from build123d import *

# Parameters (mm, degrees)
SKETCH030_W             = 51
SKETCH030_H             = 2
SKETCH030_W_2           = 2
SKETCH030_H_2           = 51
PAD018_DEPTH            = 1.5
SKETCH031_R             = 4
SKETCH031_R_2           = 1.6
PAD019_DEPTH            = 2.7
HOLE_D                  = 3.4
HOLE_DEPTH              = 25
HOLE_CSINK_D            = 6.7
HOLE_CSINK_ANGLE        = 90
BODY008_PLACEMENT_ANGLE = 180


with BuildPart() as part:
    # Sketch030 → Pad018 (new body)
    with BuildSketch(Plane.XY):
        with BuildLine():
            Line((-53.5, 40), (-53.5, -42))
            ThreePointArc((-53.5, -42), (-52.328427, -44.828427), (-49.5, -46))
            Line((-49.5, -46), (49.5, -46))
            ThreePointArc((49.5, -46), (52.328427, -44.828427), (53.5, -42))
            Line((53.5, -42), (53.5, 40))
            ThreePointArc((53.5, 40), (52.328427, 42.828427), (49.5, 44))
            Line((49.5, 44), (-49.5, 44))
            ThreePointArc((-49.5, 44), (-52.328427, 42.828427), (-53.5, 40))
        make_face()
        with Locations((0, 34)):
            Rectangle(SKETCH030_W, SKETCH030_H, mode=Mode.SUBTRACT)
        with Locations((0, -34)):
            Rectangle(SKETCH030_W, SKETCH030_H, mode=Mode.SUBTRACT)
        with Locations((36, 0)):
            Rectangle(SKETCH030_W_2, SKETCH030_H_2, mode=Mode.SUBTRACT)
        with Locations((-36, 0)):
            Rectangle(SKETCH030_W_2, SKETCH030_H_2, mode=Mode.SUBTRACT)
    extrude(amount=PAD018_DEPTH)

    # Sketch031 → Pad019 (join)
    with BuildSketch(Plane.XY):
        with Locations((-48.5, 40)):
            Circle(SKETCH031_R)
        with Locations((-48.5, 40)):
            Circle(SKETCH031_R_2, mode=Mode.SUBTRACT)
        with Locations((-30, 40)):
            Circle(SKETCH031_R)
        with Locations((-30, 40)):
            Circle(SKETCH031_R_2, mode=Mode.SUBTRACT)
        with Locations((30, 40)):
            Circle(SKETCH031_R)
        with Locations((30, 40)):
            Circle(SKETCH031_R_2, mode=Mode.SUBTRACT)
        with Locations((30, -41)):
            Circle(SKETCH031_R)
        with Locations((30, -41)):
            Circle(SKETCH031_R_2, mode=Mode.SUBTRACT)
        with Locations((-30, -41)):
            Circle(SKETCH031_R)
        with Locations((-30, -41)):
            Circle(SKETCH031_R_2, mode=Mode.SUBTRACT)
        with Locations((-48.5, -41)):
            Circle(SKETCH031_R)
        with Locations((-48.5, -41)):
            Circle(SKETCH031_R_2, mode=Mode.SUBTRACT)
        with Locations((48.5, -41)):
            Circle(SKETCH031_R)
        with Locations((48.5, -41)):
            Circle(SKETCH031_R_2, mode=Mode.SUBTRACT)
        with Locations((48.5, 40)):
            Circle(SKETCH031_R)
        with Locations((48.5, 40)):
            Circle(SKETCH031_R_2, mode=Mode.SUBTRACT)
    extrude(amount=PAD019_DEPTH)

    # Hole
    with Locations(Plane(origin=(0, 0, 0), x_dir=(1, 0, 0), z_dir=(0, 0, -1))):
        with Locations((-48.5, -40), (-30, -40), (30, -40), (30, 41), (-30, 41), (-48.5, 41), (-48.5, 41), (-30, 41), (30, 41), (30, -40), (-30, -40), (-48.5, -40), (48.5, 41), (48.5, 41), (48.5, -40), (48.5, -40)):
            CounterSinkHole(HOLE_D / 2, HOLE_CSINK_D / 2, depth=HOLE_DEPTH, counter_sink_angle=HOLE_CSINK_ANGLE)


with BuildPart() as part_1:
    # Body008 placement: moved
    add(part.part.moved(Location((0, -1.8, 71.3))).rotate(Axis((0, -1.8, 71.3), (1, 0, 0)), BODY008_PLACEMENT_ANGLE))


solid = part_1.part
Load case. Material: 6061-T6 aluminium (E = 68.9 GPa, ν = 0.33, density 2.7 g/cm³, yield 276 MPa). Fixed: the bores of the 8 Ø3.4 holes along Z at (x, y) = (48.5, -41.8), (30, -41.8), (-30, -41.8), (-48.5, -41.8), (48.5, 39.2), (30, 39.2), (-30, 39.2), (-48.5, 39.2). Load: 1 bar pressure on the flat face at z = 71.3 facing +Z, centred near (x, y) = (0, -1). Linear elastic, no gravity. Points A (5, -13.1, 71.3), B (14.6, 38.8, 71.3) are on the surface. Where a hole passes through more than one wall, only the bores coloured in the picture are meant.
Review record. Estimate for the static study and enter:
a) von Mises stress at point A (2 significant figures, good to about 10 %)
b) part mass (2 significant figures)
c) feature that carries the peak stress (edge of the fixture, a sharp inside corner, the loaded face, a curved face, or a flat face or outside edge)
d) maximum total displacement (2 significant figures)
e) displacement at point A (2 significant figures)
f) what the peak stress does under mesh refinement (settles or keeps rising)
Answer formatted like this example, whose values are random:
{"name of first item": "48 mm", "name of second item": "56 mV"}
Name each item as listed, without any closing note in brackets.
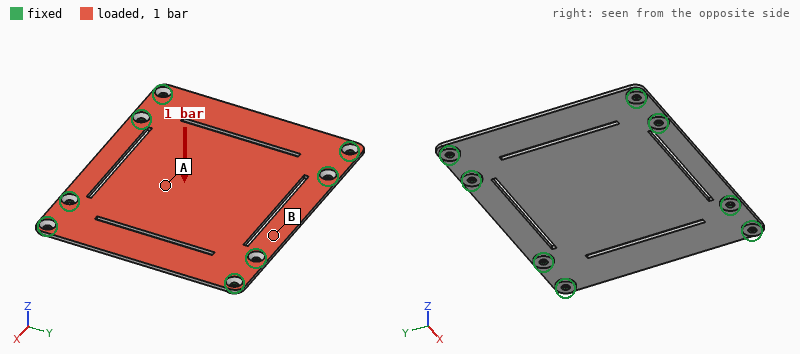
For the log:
{"von Mises stress at point A": "72 MPa", "part mass": "38 g", "feature that carries the peak stress": "edge of the fixture", "maximum total displacement": "0.97 mm", "displacement at point A": "0.88 mm", "what the peak stress does under mesh refinement": "keeps rising"}
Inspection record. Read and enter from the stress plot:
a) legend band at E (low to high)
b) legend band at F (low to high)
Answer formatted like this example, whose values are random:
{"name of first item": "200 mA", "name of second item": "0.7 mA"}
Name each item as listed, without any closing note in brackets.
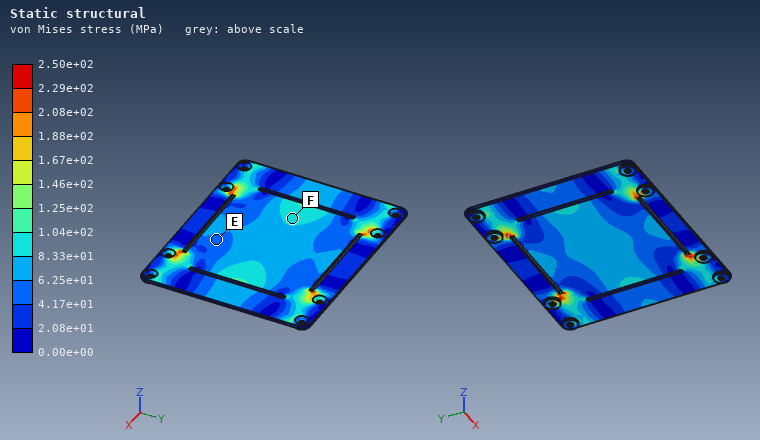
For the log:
{"legend band at E": "4.17e+01 to 6.25e+01 MPa", "legend band at F": "8.33e+01 to 1.04e+02 MPa"}
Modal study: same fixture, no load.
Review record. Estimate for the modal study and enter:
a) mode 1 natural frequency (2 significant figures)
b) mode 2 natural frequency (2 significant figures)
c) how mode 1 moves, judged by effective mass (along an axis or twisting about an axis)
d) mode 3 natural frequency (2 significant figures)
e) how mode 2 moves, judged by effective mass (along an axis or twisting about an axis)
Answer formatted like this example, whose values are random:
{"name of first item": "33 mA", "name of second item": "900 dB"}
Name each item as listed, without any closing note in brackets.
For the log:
{"mode 1 natural frequency": "960 Hz", "mode 2 natural frequency": "1400 Hz", "how mode 1 moves, judged by effective mass": "along Z", "mode 3 natural frequency": "1500 Hz", "how mode 2 moves, judged by effective mass": "twisting about Y"}
